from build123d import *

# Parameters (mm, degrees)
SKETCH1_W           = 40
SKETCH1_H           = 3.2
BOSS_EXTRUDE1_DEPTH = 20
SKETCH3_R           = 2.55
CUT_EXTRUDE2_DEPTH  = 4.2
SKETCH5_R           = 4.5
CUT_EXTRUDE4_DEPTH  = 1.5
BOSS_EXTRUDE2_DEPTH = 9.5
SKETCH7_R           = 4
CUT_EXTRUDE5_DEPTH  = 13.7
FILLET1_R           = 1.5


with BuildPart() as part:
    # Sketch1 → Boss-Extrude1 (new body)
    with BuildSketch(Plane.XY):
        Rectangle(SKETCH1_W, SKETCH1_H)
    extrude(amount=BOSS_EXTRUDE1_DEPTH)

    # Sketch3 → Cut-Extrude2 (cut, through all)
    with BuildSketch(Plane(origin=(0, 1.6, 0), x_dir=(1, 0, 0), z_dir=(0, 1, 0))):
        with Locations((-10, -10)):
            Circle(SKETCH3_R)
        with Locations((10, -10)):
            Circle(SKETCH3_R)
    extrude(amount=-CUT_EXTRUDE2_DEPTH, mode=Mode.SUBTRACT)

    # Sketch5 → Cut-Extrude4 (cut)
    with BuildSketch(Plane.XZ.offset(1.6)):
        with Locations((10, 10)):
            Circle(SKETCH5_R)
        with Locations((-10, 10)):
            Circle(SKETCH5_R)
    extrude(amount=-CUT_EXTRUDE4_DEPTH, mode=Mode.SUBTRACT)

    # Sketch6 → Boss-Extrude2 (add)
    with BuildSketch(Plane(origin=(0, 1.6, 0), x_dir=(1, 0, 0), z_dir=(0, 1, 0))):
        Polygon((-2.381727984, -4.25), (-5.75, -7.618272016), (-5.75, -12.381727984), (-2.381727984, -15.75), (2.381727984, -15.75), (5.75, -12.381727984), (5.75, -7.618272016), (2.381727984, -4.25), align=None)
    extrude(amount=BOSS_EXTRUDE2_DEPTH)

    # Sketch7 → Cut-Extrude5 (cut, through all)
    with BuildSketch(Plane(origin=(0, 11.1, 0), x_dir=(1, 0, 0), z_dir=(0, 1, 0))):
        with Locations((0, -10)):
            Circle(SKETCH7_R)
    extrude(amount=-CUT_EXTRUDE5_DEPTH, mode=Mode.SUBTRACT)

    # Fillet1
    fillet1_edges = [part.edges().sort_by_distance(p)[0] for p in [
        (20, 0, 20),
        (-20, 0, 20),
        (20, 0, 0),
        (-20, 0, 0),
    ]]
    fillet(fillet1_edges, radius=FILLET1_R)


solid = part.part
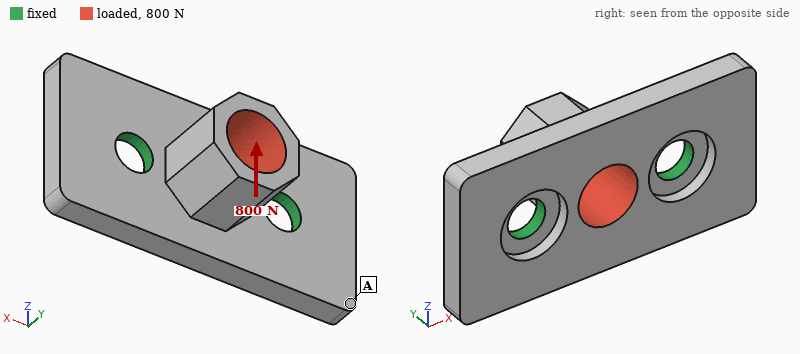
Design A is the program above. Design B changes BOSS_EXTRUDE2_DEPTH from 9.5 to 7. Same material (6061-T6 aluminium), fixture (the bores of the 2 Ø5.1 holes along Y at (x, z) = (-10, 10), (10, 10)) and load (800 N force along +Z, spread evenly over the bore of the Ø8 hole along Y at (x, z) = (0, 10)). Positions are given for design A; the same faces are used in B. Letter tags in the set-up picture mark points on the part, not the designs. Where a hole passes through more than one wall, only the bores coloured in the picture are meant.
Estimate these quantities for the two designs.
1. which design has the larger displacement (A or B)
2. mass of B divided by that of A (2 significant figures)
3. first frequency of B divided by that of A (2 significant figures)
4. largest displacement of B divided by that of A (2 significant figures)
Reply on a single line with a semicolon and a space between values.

A; 0.95; 1.1; 0.59
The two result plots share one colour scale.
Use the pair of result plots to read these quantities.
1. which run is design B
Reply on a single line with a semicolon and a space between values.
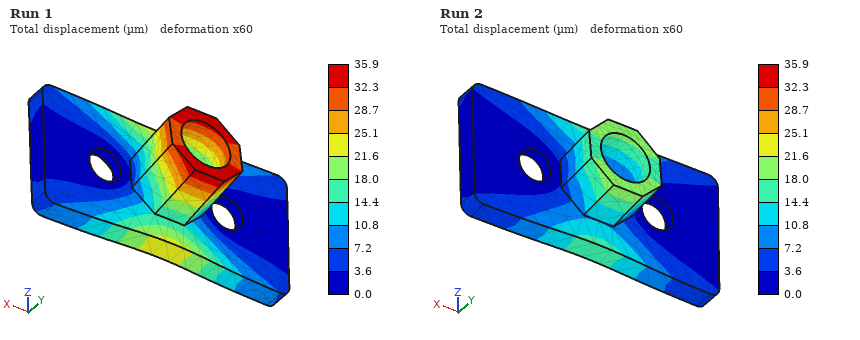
Run 2
